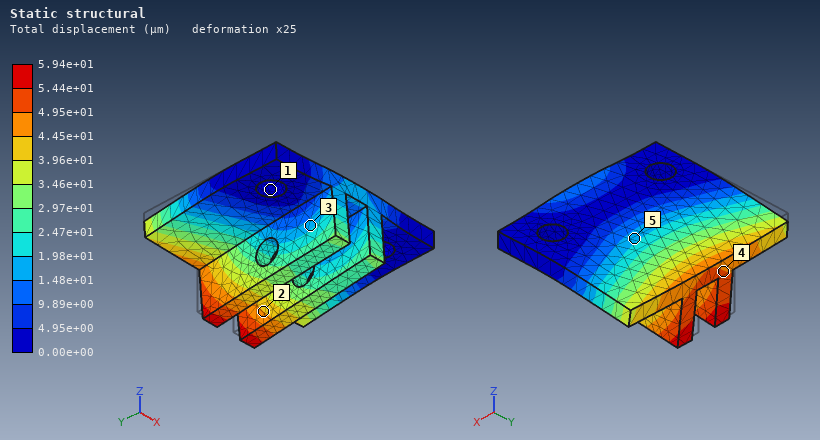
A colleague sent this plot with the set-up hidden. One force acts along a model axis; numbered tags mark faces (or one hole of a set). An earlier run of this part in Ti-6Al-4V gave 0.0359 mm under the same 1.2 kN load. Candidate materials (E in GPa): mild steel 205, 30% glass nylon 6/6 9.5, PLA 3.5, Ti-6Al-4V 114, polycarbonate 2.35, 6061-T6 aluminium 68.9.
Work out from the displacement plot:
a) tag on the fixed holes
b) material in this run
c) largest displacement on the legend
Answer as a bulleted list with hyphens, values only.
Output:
- 1
- 6061-T6 aluminium
- 5.94e+01 µm
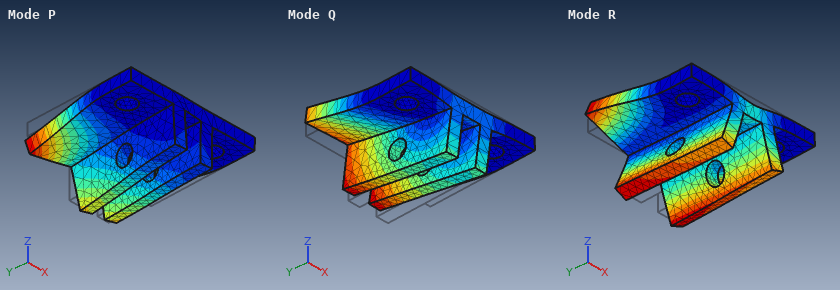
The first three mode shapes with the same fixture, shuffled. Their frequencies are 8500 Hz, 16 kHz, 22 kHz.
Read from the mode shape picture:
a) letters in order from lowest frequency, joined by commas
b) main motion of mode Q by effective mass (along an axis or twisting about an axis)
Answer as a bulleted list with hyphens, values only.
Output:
- Q, P, R
- along Z
